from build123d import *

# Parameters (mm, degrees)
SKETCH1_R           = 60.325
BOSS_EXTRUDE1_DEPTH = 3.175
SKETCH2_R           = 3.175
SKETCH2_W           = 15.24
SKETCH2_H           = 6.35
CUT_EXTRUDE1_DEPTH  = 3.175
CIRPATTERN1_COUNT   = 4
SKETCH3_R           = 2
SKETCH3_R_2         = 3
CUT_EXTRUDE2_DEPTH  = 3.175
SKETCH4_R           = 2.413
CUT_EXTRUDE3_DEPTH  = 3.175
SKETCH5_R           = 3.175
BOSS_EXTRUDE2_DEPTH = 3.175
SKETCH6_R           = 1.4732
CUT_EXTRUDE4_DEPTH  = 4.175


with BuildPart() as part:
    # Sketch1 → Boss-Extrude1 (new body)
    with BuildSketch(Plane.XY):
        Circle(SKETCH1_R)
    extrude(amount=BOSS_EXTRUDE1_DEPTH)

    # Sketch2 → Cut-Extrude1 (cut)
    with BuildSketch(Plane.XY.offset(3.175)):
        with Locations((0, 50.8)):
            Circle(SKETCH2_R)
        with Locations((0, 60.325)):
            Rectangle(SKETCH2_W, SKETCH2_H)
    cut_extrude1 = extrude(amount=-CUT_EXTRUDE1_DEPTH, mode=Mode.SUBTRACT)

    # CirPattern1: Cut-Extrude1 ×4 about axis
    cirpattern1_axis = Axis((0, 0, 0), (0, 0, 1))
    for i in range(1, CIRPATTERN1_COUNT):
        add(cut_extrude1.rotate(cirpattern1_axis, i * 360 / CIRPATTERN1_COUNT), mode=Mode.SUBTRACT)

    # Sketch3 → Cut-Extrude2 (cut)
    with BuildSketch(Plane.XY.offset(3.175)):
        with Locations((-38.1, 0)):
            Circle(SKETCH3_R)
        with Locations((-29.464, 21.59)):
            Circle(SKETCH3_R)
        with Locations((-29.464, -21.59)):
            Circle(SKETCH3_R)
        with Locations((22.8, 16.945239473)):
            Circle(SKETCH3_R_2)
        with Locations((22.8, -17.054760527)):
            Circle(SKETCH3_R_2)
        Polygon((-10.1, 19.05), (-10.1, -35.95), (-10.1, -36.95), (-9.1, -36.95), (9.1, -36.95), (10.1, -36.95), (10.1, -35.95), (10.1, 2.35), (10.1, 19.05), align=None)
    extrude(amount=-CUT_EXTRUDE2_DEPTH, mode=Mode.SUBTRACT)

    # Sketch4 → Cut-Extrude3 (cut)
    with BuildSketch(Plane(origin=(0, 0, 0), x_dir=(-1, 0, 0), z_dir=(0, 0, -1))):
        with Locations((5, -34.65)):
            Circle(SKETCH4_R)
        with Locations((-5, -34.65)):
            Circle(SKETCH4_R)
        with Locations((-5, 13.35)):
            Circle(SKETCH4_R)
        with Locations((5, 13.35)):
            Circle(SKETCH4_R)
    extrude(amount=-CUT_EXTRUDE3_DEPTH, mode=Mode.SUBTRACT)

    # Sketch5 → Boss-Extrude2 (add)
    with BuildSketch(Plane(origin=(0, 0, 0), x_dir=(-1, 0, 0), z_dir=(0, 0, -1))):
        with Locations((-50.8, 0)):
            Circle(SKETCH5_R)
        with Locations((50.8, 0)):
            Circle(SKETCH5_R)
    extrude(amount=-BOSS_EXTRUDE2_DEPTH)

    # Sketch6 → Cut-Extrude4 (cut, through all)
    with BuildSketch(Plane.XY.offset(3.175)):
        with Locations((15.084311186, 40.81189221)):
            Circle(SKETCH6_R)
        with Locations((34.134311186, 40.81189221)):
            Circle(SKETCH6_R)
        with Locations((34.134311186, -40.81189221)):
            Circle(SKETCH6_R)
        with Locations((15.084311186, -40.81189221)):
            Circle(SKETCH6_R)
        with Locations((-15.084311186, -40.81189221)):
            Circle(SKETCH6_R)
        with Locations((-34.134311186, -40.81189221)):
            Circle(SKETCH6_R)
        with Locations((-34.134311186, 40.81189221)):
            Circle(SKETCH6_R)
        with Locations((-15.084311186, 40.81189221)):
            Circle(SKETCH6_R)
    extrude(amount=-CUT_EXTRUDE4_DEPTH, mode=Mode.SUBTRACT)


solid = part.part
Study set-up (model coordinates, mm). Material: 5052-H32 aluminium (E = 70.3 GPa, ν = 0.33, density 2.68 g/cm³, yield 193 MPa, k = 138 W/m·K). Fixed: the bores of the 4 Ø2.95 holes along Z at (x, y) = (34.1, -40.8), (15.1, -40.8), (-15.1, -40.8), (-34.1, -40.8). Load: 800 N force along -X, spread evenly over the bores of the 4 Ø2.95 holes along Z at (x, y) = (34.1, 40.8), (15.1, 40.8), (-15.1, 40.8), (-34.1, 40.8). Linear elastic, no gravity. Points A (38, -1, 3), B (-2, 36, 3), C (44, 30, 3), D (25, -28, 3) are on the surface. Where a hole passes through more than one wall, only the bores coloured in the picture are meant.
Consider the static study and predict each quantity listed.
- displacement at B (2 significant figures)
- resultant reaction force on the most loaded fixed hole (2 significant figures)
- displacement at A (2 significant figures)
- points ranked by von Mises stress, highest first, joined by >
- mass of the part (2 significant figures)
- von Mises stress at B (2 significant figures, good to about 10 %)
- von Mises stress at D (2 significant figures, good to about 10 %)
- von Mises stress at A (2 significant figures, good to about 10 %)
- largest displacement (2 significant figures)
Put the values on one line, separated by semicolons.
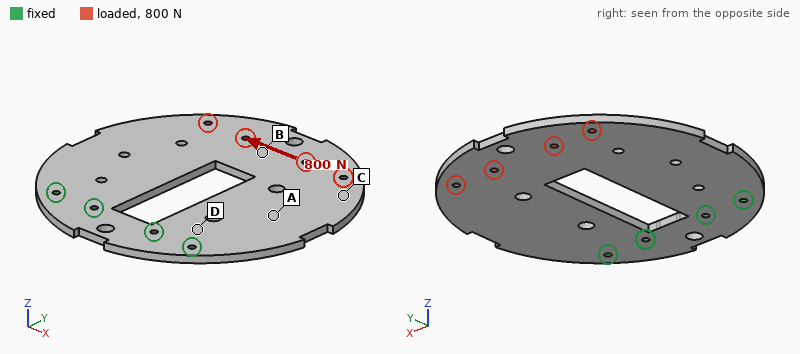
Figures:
43 µm; 1.1 kN; 26 µm; D > B > A > C; 84 g; 13 MPa; 16 MPa; 6.5 MPa; 50 µm
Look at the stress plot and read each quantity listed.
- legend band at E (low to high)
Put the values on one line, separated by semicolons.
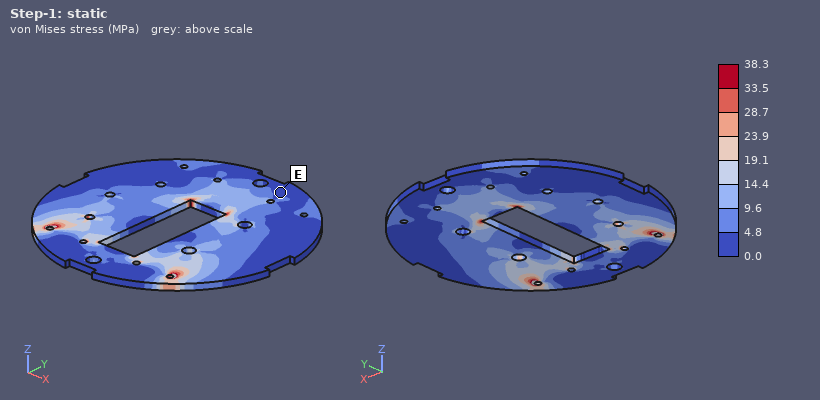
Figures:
0.0 to 4.8 MPa
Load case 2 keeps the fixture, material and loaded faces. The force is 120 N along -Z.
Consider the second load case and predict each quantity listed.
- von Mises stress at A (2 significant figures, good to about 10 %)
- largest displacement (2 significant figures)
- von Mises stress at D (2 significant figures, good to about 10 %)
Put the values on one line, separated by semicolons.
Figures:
30 MPa; 1.9 mm; 56 MPa
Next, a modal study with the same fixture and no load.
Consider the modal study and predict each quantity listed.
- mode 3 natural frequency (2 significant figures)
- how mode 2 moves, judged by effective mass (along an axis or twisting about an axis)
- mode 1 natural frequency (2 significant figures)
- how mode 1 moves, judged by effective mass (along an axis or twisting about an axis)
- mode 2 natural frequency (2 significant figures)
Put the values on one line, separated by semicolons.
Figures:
1400 Hz; twisting about Y; 270 Hz; along Z; 640 Hz
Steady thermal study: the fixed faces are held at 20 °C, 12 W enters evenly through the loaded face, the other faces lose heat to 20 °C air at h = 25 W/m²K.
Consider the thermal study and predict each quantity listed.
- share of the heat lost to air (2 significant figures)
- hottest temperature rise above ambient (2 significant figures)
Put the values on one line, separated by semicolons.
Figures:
42 %; 20 K
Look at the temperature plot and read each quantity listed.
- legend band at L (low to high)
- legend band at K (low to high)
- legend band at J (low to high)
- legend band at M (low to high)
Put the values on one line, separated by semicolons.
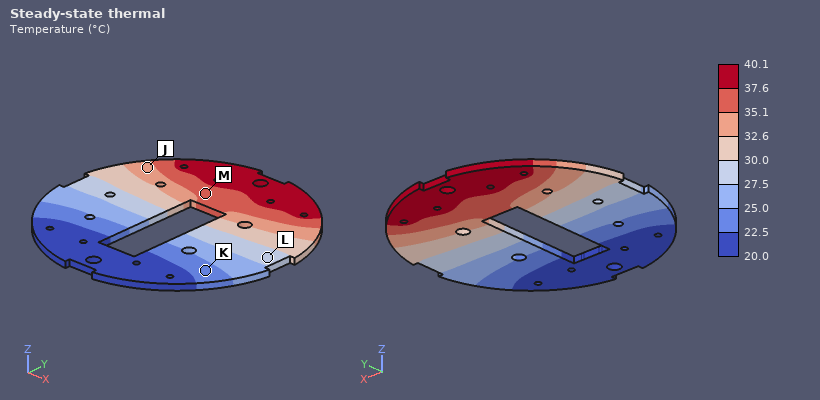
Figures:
27.5 to 30.0 °C; 22.5 to 25.0 °C; 32.6 to 35.1 °C; 35.1 to 37.6 °C
